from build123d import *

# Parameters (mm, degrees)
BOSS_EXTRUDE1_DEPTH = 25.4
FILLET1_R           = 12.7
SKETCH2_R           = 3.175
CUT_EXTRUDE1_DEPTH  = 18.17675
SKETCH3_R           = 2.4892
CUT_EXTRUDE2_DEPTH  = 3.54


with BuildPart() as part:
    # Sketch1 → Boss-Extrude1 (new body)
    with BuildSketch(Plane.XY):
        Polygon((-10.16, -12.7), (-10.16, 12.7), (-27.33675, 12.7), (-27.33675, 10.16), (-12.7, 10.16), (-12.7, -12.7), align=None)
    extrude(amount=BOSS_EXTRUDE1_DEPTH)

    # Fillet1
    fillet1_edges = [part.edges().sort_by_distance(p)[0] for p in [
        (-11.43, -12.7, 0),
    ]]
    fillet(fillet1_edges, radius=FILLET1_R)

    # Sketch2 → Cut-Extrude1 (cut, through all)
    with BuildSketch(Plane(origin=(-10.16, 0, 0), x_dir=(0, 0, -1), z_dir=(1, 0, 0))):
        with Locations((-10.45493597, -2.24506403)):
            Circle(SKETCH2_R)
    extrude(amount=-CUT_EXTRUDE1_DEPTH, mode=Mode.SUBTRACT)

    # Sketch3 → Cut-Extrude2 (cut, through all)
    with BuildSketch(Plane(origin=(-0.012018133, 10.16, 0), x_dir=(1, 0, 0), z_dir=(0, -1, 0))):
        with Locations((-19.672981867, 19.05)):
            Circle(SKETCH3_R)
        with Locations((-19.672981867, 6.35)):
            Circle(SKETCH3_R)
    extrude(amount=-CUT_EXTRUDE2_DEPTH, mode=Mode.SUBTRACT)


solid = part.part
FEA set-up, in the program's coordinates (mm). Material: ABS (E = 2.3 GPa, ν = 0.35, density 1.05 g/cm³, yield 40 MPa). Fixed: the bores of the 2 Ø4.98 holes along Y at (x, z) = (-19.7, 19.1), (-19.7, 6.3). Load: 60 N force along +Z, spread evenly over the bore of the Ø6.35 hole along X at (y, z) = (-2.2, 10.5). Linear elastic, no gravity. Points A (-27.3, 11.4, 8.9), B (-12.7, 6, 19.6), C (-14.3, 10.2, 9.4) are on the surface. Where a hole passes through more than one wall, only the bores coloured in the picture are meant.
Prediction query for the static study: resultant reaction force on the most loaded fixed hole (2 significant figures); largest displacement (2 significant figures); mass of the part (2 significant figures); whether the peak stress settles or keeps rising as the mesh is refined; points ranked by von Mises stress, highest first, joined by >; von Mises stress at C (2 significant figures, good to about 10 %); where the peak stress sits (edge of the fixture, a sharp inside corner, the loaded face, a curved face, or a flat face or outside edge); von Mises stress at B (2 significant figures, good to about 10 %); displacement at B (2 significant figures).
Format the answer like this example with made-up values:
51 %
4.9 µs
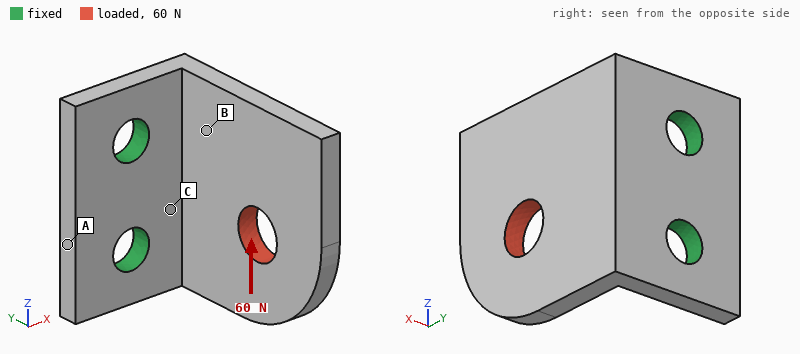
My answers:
64 N
0.38 mm
2.4 g
keeps rising
C > B > A
9.3 MPa
edge of the fixture
5.6 MPa
0.11 mm
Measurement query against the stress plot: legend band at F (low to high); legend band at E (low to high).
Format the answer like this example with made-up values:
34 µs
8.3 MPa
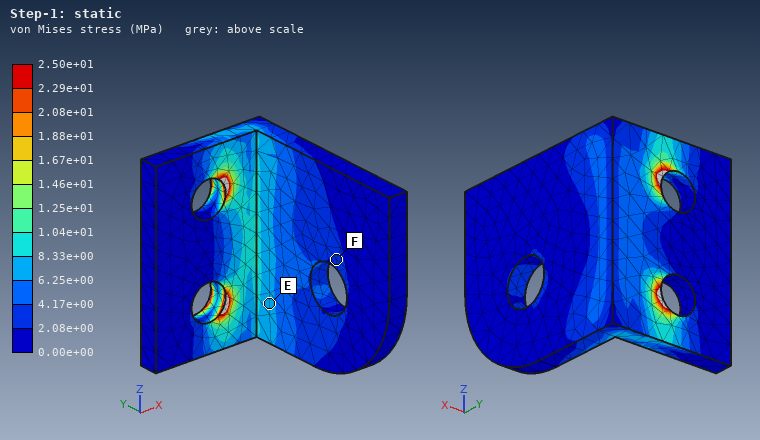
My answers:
2.08e+00 to 4.17e+00 MPa
6.25e+00 to 8.33e+00 MPa
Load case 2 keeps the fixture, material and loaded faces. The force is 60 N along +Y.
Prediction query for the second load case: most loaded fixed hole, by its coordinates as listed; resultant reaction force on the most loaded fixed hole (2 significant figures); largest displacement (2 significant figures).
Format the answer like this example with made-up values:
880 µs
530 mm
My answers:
(-19.7, 6.3)
38 N
0.41 mm
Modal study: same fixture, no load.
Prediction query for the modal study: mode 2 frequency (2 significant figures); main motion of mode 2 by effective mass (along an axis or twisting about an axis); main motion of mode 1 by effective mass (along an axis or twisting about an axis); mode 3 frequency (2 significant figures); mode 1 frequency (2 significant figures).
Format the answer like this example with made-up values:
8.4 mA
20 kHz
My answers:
2000 Hz
along Z
along X
2800 Hz
840 Hz
